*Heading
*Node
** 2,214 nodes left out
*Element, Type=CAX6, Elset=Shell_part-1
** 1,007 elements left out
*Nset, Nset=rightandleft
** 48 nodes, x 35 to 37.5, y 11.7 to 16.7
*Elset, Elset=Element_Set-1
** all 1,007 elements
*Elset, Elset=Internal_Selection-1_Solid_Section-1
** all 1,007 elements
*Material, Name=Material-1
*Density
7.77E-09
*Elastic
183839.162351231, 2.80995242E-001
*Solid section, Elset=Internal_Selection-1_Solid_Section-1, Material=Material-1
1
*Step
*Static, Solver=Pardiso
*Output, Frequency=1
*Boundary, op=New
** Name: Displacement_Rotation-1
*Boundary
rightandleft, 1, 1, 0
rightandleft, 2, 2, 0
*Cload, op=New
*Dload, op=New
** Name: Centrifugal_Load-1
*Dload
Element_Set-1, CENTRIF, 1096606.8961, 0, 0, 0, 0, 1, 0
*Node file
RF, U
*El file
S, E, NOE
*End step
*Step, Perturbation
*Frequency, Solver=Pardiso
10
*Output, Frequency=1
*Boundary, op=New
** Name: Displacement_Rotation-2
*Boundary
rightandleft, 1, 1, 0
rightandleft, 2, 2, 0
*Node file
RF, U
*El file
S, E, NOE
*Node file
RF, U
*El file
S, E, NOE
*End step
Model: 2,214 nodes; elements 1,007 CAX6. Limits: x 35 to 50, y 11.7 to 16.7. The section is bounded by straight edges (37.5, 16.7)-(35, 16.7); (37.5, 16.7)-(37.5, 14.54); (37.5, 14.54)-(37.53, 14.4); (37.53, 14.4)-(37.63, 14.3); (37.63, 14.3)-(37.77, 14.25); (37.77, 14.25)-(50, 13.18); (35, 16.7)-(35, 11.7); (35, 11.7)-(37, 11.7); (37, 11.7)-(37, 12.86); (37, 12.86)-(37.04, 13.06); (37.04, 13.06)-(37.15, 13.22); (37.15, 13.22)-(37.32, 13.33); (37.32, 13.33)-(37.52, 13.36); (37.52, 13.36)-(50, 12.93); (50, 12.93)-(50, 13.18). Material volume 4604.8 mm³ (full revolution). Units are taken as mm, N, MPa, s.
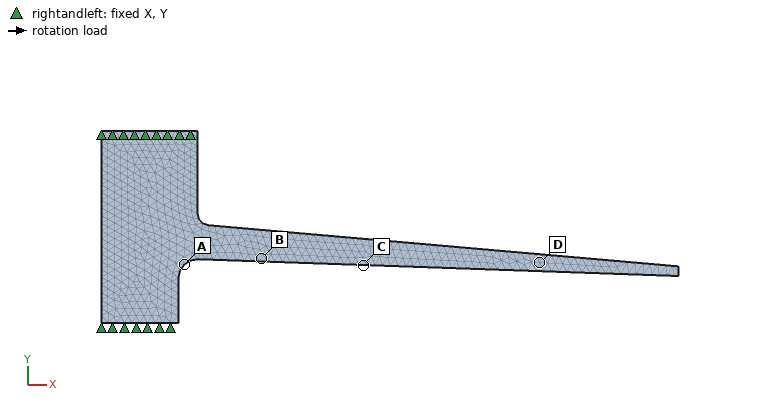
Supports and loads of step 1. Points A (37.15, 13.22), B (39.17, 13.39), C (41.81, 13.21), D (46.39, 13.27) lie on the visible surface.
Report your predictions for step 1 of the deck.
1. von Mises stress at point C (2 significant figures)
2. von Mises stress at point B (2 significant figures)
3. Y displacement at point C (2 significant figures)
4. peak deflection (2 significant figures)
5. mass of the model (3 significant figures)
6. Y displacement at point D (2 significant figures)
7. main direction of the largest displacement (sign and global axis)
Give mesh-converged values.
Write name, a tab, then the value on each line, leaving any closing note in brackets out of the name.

von Mises stress at point C	5.5 MPa
von Mises stress at point B	6.3 MPa
Y displacement at point C	8.0e-04 mm
peak deflection	0.0049 mm
mass of the model	0.0358 kg
Y displacement at point D	0.0028 mm
main direction of the largest displacement	+Y
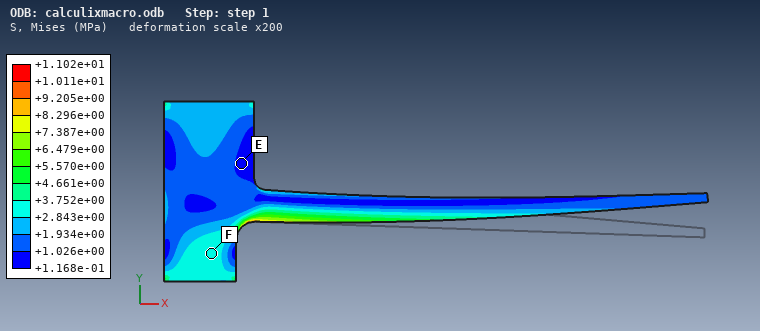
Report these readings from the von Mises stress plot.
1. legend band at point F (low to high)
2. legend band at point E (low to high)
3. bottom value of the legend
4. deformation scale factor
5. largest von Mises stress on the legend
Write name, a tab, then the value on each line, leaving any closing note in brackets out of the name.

legend band at point F	+2.843e+00 to +3.752e+00 MPa
legend band at point E	+1.168e-01 to +1.026e+00 MPa
bottom value of the legend	+1.168e-01 MPa
deformation scale factor	200
largest von Mises stress on the legend	+1.102e+01 MPa
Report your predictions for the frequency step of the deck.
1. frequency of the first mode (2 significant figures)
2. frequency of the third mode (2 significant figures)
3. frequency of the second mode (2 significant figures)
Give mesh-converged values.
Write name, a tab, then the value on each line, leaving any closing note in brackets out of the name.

frequency of the first mode	5200 Hz
frequency of the third mode	50000 Hz
frequency of the second mode	21000 Hz
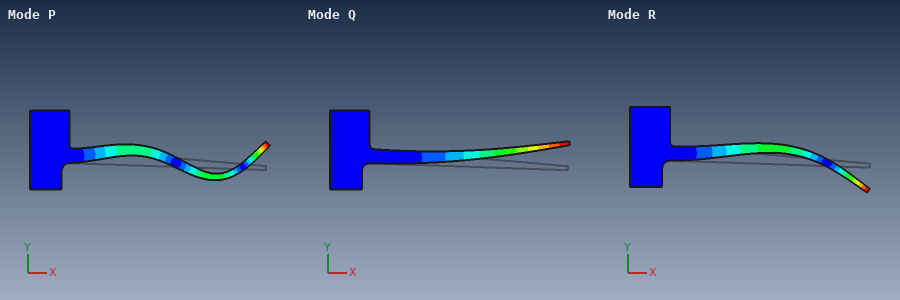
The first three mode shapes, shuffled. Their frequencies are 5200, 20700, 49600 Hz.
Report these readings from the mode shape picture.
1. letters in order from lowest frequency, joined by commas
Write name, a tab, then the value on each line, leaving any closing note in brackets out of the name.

letters in order from lowest frequency, joined by commas	Q, R, P
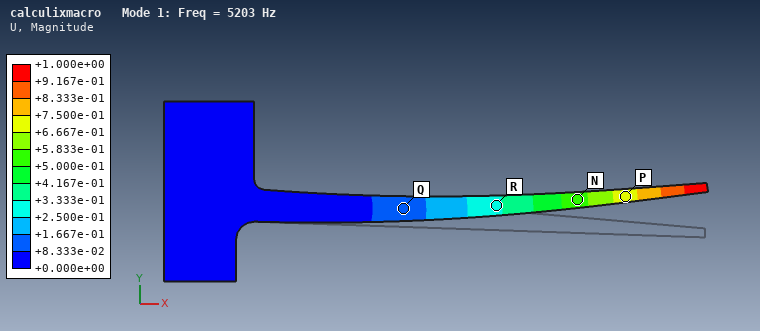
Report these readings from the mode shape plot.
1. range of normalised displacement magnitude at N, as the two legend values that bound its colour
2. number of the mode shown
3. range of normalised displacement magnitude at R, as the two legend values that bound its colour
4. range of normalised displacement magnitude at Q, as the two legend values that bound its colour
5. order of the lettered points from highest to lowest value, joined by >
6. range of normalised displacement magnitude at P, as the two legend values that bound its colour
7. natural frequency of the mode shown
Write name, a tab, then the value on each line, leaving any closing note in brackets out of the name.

range of normalised displacement magnitude at N, as the two legend values that bound its colour	+5.000e-01 to +5.833e-01
number of the mode shown	1
range of normalised displacement magnitude at R, as the two legend values that bound its colour	+2.500e-01 to +3.333e-01
range of normalised displacement magnitude at Q, as the two legend values that bound its colour	+8.333e-02 to +1.667e-01
order of the lettered points from highest to lowest value, joined by >	P > N > R > Q
range of normalised displacement magnitude at P, as the two legend values that bound its colour	+6.667e-01 to +7.500e-01
natural frequency of the mode shown	5203 Hz
